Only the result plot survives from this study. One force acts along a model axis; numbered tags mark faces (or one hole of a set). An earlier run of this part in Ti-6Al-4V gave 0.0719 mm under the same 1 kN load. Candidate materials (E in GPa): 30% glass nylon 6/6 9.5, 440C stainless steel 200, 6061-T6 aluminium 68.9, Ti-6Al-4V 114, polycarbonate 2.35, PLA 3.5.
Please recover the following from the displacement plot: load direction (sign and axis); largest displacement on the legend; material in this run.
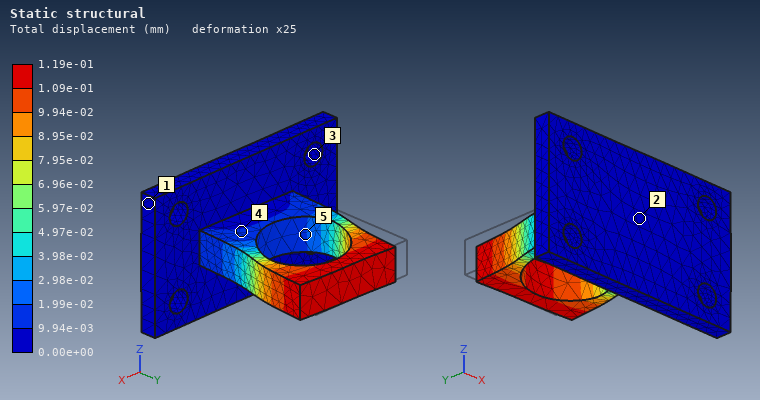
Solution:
+X
1.19e-01 mm
6061-T6 aluminium
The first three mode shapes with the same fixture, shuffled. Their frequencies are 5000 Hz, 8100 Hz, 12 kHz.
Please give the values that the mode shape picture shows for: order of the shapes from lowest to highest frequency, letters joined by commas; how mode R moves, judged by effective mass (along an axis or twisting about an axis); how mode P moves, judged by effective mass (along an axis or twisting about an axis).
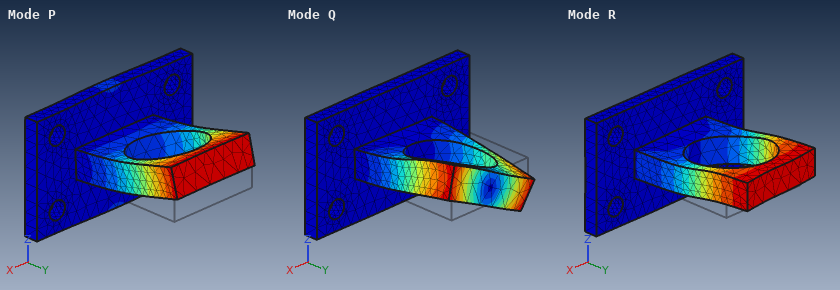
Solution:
P, R, Q
along X
along Z
